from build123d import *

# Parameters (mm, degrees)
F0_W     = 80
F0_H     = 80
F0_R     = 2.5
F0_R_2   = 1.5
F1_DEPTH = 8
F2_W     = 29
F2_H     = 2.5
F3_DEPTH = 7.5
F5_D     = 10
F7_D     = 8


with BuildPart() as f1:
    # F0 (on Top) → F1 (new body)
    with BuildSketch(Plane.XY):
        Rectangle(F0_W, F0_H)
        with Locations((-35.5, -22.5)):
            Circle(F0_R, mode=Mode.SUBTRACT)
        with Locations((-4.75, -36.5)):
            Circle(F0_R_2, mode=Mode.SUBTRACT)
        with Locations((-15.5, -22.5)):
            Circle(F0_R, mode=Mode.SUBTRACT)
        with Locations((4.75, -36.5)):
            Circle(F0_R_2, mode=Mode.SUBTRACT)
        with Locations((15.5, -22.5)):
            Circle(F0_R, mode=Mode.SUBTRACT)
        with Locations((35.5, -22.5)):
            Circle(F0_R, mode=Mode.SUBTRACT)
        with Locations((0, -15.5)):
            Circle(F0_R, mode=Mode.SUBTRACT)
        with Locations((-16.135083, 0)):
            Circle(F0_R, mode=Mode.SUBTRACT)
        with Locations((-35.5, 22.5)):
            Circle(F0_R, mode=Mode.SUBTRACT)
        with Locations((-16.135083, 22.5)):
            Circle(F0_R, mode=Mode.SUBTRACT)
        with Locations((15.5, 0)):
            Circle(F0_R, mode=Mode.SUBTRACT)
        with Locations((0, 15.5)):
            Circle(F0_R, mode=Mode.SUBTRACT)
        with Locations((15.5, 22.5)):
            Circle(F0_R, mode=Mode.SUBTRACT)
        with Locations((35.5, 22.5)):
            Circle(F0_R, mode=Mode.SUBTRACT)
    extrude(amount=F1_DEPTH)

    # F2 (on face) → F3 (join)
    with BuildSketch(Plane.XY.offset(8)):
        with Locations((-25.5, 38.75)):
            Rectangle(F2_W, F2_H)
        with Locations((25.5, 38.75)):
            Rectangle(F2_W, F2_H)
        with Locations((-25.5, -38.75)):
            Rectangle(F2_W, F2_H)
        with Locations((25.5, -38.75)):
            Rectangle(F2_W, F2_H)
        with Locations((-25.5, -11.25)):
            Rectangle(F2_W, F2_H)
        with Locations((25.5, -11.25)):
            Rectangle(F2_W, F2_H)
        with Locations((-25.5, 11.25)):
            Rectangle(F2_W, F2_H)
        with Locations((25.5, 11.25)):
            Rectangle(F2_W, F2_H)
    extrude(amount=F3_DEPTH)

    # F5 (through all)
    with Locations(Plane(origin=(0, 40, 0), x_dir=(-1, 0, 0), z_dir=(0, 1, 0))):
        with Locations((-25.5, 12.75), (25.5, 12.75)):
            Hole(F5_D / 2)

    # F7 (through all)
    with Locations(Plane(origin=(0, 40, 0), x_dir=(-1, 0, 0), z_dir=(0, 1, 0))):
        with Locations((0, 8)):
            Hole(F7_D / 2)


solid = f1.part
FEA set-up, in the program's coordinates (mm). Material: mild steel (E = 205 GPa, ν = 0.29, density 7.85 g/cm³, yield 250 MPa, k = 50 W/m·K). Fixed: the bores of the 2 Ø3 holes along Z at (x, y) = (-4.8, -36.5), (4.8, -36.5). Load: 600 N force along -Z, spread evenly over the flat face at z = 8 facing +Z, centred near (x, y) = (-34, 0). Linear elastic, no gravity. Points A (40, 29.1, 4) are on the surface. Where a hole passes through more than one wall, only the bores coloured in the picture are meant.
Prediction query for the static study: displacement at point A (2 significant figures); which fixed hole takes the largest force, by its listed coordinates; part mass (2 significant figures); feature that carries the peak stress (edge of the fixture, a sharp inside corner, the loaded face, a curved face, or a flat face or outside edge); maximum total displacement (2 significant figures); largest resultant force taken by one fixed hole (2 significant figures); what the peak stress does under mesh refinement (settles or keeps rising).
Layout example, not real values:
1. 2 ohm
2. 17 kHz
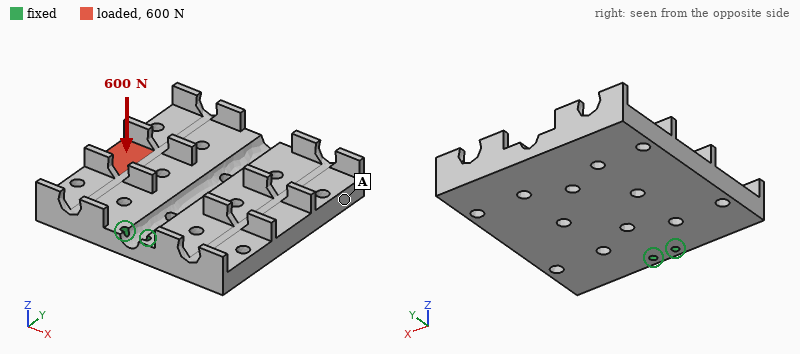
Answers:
1. 0.034 mm
2. (-4.8, -36.5)
3. 390 g
4. edge of the fixture
5. 0.16 mm
6. 1.0 kN
7. keeps rising
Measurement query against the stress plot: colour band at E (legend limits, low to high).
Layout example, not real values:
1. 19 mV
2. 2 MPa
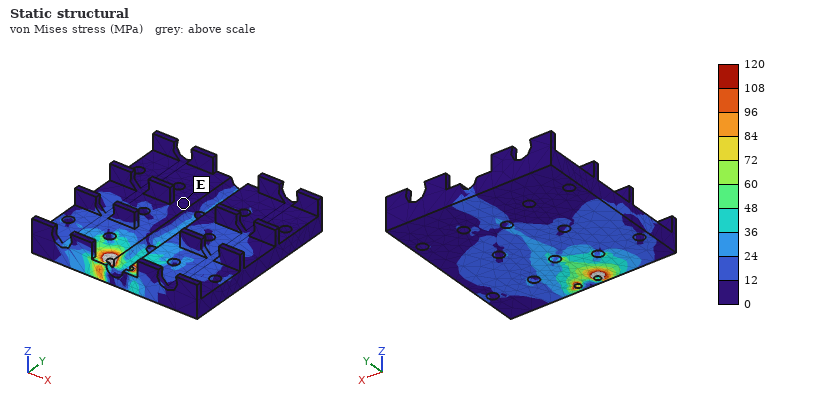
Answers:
1. 0 to 12 MPa
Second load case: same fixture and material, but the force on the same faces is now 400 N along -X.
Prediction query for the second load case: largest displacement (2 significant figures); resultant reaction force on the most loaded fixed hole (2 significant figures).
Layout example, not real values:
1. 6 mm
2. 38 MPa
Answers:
1. 21 µm
2. 1.1 kN
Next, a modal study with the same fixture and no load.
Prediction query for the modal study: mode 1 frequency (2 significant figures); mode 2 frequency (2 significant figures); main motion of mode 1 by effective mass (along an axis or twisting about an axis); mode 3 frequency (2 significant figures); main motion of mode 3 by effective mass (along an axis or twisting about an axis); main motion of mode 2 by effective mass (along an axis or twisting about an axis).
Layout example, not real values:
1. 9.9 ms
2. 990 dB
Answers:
1. 730 Hz
2. 1300 Hz
3. along Z
4. 1500 Hz
5. along X
6. along X
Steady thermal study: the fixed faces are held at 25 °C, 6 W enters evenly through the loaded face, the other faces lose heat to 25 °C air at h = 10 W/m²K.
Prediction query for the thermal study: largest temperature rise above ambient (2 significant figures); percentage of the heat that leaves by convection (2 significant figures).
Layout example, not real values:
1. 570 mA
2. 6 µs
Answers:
1. 17 K
2. 25 %
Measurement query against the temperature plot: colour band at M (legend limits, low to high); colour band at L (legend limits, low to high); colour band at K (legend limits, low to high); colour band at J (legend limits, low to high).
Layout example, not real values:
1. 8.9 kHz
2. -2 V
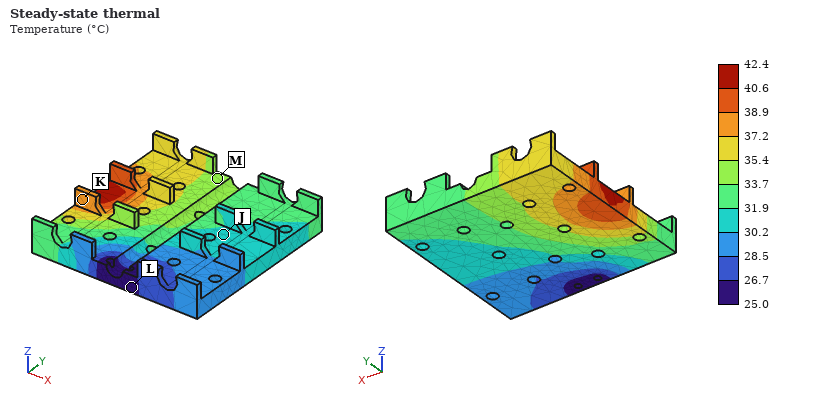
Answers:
1. 33.7 to 35.4 °C
2. 25.0 to 26.7 °C
3. 37.2 to 38.9 °C
4. 30.2 to 31.9 °C
